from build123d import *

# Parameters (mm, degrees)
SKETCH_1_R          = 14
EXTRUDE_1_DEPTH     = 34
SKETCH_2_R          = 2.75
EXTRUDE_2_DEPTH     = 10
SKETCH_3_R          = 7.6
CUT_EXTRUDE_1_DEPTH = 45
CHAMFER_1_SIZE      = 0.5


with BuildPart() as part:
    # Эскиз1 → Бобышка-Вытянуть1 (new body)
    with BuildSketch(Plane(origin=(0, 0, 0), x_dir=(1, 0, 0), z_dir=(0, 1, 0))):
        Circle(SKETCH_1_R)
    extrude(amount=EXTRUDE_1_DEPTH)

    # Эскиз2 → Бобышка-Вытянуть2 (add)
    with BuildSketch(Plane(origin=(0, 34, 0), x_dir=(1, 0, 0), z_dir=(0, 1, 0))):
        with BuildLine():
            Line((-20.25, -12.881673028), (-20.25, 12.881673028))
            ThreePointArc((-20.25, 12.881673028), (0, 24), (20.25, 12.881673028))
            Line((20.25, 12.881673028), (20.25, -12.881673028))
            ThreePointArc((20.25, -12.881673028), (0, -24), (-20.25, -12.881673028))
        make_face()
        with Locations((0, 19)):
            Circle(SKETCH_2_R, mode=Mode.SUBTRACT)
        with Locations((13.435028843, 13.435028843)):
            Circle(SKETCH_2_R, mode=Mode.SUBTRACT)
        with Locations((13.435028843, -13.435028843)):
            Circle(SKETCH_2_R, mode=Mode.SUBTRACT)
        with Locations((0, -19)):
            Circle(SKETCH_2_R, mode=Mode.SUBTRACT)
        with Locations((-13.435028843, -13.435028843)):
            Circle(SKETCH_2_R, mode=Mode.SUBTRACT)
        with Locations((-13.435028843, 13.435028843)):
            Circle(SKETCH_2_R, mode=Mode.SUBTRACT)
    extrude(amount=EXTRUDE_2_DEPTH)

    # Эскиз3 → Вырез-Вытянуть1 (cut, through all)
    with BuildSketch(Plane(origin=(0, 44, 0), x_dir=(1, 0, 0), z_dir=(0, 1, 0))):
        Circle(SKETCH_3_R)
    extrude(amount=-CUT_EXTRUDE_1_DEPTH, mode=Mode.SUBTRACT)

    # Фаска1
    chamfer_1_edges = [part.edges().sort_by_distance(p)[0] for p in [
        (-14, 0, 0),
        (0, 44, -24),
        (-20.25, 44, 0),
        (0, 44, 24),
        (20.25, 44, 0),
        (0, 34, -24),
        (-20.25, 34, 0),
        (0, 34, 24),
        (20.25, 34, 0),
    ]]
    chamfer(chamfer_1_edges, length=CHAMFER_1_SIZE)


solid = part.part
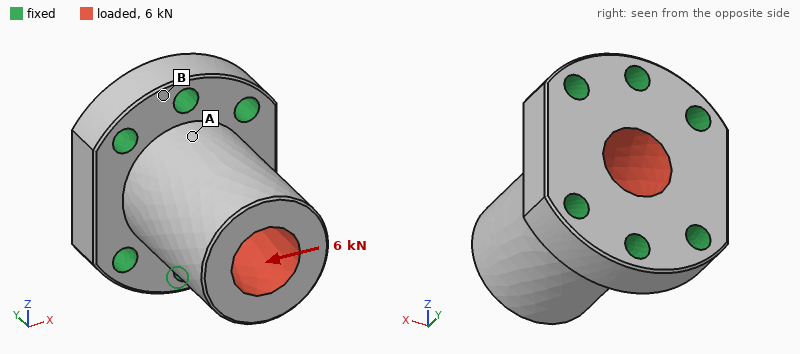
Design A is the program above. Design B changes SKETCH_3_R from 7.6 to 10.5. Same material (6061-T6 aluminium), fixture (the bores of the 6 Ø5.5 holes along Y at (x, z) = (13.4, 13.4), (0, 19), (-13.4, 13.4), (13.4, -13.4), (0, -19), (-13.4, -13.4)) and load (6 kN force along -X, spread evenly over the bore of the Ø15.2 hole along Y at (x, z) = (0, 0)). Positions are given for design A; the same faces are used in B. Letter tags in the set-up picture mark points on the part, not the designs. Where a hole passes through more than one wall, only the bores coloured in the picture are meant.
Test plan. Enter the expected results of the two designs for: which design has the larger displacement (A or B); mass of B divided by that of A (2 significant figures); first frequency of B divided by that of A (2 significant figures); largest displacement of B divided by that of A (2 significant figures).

B
0.74
1.1
1.4
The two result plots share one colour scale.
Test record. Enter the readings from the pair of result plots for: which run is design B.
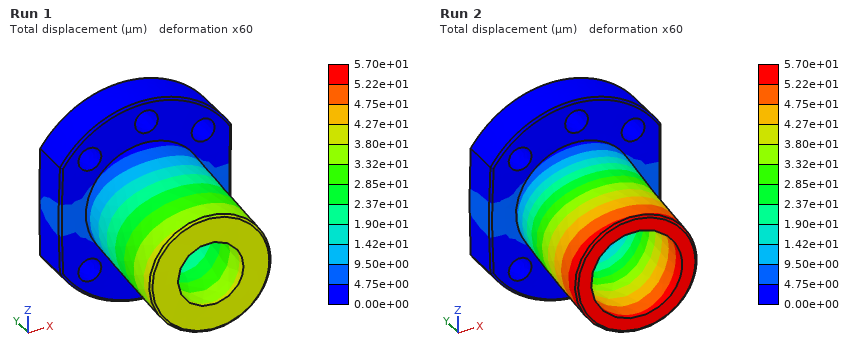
Run 2
